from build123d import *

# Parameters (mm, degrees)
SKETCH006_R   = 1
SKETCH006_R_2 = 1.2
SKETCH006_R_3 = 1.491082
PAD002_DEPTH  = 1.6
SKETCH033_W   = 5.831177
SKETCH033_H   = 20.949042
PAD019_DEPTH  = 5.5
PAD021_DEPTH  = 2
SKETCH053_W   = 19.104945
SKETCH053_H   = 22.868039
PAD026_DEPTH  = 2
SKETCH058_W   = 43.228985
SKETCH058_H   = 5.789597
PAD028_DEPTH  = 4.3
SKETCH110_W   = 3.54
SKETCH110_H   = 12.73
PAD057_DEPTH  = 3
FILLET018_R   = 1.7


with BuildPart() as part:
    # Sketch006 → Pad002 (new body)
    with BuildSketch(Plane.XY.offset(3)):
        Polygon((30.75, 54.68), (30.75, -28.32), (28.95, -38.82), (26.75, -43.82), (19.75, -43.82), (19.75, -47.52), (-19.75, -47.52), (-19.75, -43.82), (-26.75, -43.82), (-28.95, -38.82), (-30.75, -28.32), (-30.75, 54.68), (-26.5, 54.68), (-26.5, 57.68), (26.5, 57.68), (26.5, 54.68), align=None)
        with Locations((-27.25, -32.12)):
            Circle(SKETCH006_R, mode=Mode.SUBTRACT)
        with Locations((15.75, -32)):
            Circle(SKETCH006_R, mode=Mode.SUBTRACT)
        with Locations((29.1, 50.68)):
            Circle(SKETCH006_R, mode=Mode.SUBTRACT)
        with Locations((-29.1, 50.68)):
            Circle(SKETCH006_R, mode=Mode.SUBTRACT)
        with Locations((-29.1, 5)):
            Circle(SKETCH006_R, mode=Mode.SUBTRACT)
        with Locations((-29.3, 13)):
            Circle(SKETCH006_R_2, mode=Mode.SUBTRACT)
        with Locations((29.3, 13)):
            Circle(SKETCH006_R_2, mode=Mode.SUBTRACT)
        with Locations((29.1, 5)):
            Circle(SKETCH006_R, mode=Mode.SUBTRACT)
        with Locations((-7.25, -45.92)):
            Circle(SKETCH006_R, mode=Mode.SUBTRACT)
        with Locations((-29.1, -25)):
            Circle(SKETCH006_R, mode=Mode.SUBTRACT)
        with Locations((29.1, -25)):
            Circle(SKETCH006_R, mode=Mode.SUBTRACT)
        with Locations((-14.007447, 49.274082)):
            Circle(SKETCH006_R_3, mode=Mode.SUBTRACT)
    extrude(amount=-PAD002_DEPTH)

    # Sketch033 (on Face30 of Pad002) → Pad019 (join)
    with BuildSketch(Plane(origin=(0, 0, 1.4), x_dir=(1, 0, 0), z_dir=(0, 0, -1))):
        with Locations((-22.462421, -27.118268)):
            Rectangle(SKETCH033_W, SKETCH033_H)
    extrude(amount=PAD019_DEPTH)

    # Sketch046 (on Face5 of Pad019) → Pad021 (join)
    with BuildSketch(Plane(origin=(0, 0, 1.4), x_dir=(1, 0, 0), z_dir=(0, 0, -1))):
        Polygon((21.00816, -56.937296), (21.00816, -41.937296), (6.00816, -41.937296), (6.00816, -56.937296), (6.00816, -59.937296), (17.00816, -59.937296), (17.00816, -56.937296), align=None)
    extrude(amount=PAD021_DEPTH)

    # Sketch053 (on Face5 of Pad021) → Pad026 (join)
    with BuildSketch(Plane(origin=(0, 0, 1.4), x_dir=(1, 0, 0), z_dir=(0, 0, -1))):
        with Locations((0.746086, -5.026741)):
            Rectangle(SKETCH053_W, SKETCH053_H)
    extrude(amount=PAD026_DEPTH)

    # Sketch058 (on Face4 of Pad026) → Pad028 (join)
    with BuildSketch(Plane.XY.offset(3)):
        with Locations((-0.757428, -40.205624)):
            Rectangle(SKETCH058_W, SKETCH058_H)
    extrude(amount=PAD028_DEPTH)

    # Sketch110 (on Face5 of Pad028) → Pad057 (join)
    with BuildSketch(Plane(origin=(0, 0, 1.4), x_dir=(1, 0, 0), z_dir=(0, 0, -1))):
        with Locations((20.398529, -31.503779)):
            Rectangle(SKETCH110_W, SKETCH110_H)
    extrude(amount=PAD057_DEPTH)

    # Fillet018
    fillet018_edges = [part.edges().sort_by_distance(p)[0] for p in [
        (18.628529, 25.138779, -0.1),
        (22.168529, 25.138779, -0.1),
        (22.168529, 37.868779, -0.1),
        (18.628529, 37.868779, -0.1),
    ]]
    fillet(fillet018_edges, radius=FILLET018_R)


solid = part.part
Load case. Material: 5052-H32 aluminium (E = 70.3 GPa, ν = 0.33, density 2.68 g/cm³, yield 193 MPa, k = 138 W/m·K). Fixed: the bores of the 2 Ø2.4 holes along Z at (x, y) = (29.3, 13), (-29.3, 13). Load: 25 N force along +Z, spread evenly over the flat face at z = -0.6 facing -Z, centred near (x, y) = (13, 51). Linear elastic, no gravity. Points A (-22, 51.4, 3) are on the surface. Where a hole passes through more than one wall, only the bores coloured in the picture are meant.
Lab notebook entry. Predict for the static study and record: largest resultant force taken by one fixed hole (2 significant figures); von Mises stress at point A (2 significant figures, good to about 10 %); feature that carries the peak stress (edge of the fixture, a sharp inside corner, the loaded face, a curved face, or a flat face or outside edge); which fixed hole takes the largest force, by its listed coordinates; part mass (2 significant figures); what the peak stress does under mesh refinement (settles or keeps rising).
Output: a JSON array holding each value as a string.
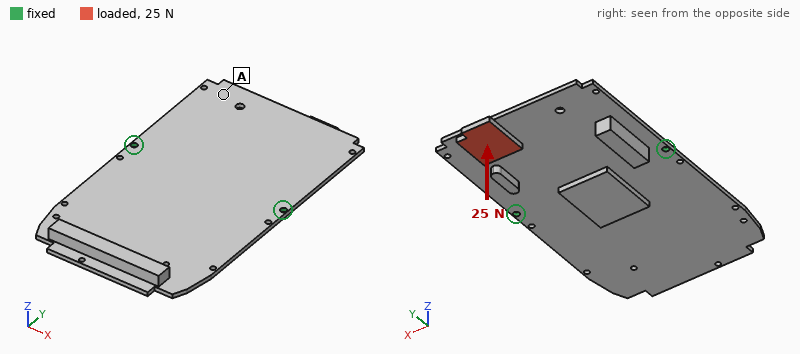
["20 N", "8.2 MPa", "edge of the fixture", "(29.3, 13)", "36 g", "keeps rising"]
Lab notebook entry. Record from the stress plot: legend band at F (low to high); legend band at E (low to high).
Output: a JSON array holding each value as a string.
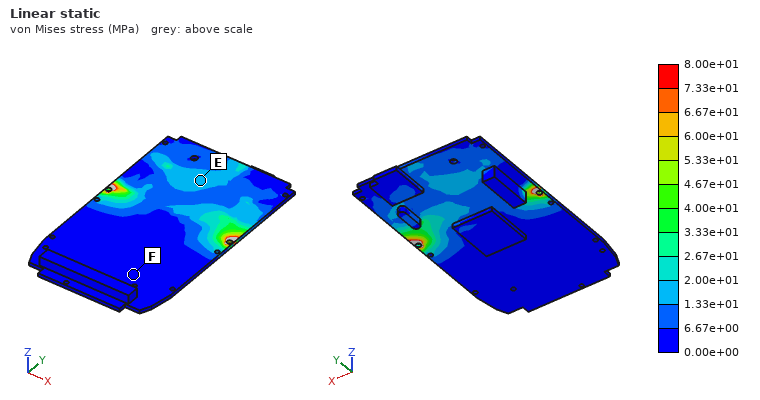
["0.00e+00 to 6.67e+00 MPa", "1.33e+01 to 2.00e+01 MPa"]
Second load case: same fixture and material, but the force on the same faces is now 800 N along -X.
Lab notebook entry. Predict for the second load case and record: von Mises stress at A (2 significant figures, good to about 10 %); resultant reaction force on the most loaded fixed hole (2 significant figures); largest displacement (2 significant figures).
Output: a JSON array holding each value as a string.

["13 MPa", "670 N", "0.48 mm"]
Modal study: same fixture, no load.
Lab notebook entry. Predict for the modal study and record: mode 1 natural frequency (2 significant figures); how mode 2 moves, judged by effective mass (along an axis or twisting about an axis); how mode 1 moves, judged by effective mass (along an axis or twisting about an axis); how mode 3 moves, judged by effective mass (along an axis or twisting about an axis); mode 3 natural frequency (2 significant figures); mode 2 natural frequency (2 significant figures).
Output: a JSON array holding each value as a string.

["260 Hz", "along Z", "along Z", "twisting about Y", "1100 Hz", "620 Hz"]
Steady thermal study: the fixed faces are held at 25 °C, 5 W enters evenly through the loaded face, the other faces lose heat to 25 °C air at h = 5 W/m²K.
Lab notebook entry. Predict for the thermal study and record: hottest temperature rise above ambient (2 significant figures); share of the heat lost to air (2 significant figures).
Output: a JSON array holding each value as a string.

["21 K", "11 %"]
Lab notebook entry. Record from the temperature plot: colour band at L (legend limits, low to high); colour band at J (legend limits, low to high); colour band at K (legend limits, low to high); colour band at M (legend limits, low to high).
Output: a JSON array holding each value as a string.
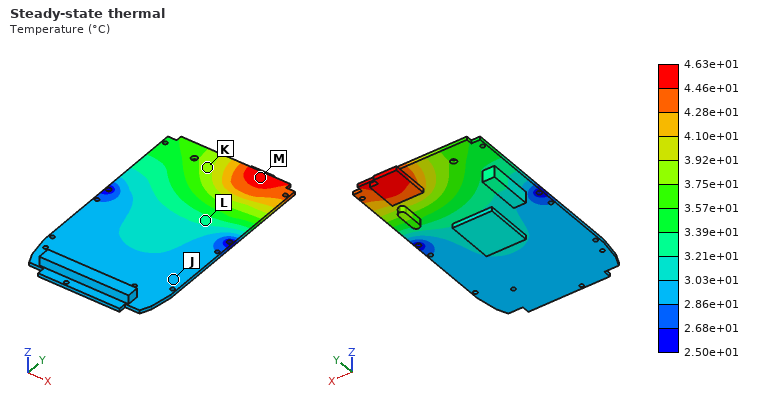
["3.21e+01 to 3.39e+01 °C", "2.86e+01 to 3.03e+01 °C", "3.75e+01 to 3.92e+01 °C", "4.46e+01 to 4.63e+01 °C"]
